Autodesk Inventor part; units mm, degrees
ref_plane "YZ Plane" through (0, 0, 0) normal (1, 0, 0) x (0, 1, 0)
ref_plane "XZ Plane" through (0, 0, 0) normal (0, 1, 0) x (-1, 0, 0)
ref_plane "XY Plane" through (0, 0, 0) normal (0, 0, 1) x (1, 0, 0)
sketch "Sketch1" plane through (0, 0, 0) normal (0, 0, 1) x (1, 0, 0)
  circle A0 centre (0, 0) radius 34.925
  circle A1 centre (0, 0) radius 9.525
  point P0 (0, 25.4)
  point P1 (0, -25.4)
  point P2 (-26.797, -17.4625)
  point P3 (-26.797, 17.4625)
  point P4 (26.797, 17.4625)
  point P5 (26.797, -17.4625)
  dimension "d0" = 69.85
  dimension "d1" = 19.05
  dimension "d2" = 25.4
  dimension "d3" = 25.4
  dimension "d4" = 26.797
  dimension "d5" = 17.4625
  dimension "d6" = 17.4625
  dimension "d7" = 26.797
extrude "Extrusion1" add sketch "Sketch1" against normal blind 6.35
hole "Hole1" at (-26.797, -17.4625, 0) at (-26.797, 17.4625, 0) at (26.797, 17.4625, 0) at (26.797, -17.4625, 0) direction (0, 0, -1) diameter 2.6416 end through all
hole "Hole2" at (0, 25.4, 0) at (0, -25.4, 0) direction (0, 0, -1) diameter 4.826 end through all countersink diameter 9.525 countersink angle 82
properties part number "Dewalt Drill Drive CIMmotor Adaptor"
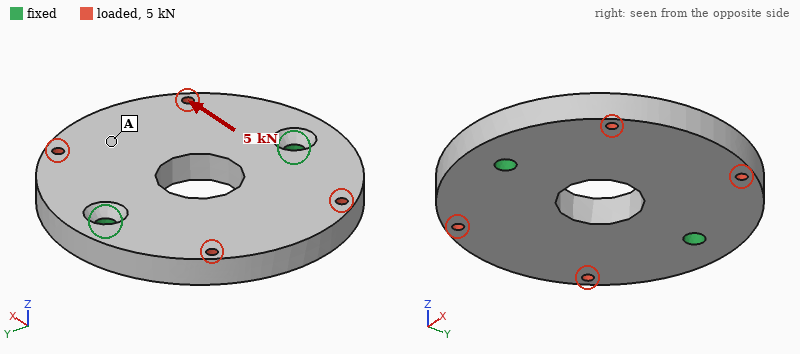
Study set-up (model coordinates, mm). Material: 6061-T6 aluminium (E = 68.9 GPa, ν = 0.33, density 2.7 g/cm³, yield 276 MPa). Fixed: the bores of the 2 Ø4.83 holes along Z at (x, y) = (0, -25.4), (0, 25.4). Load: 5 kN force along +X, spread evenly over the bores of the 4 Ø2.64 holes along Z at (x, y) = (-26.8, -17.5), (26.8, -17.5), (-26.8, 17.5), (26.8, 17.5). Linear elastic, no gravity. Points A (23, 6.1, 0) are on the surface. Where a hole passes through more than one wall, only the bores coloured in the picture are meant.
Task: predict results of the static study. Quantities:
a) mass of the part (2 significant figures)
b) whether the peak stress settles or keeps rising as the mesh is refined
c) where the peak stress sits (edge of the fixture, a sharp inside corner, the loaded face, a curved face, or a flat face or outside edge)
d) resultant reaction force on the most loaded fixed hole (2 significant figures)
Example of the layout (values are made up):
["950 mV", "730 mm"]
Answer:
["59 g", "keeps rising", "edge of the fixture", "2.5 kN"]
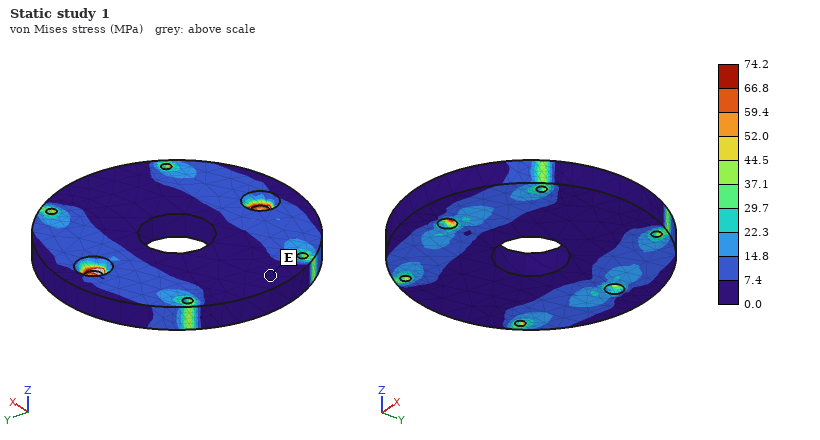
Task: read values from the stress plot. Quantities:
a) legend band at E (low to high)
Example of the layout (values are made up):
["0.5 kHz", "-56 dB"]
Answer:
["0.0 to 7.4 MPa"]
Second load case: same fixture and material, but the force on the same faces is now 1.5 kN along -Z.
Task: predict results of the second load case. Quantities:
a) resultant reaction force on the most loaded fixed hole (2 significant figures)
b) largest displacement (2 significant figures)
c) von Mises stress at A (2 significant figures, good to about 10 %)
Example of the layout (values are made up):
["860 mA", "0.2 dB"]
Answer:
["800 N", "0.11 mm", "11 MPa"]
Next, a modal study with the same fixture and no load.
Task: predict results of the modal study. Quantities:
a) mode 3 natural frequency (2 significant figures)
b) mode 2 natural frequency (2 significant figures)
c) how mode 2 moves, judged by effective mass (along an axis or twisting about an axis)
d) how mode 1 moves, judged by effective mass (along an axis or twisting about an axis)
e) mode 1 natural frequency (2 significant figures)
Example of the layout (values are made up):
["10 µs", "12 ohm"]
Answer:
["8400 Hz", "4200 Hz", "along Z", "twisting about Y", "3000 Hz"]
